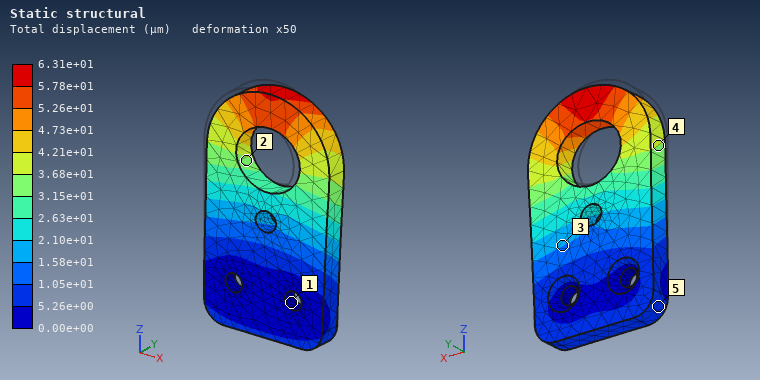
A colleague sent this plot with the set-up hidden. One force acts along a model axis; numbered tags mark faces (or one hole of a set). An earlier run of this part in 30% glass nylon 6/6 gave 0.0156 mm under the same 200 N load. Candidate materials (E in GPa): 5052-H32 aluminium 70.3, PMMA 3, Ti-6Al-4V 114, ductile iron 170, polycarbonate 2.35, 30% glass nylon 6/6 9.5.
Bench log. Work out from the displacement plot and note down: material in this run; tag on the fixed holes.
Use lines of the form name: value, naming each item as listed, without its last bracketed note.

material in this run: polycarbonate
tag on the fixed holes: 1
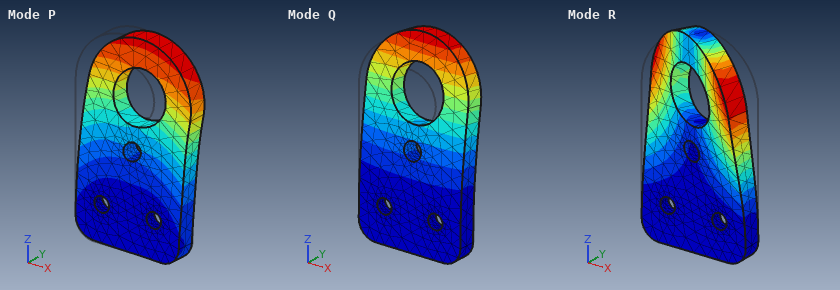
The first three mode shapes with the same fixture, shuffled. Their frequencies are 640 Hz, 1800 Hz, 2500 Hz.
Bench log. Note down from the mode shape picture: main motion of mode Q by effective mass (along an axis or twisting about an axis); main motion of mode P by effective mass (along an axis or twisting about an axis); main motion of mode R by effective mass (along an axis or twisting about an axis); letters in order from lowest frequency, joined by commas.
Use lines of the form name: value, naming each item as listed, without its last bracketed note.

main motion of mode Q by effective mass: along Y
main motion of mode P by effective mass: along X
main motion of mode R by effective mass: twisting about Z
letters in order from lowest frequency, joined by commas: Q, R, P
